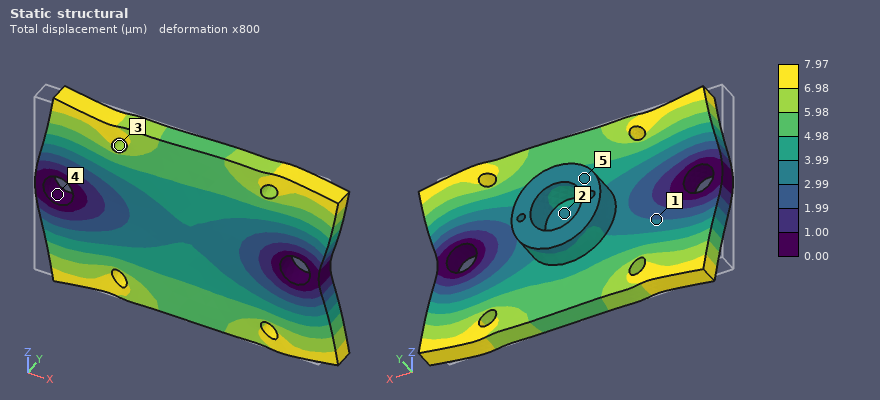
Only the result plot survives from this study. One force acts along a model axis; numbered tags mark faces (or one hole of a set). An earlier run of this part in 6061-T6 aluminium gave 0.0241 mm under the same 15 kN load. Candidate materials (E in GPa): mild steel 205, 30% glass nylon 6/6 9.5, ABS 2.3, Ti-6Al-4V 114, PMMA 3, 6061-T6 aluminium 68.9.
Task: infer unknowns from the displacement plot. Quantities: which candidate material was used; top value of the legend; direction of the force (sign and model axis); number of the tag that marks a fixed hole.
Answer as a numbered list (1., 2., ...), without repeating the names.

1. mild steel
2. 7.97 µm
3. +X
4. 4
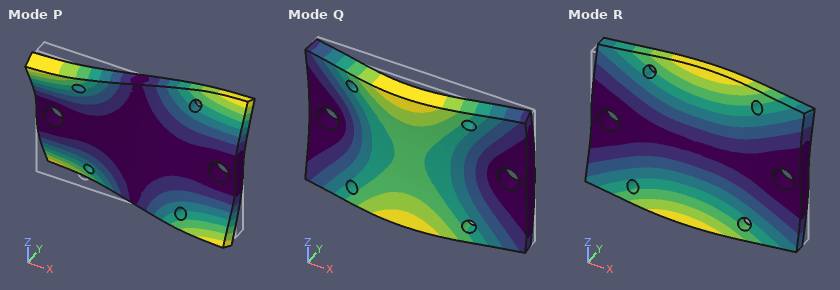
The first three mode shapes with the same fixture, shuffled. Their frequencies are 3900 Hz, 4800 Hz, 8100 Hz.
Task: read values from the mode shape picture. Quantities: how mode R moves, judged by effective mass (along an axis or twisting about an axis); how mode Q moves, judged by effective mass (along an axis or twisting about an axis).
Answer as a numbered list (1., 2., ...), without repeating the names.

1. twisting about X
2. along Y
